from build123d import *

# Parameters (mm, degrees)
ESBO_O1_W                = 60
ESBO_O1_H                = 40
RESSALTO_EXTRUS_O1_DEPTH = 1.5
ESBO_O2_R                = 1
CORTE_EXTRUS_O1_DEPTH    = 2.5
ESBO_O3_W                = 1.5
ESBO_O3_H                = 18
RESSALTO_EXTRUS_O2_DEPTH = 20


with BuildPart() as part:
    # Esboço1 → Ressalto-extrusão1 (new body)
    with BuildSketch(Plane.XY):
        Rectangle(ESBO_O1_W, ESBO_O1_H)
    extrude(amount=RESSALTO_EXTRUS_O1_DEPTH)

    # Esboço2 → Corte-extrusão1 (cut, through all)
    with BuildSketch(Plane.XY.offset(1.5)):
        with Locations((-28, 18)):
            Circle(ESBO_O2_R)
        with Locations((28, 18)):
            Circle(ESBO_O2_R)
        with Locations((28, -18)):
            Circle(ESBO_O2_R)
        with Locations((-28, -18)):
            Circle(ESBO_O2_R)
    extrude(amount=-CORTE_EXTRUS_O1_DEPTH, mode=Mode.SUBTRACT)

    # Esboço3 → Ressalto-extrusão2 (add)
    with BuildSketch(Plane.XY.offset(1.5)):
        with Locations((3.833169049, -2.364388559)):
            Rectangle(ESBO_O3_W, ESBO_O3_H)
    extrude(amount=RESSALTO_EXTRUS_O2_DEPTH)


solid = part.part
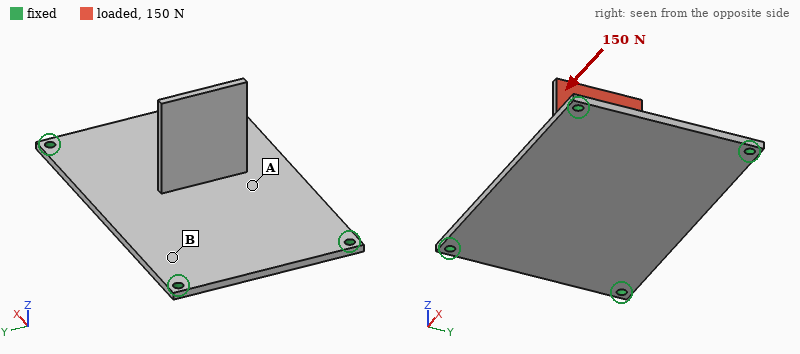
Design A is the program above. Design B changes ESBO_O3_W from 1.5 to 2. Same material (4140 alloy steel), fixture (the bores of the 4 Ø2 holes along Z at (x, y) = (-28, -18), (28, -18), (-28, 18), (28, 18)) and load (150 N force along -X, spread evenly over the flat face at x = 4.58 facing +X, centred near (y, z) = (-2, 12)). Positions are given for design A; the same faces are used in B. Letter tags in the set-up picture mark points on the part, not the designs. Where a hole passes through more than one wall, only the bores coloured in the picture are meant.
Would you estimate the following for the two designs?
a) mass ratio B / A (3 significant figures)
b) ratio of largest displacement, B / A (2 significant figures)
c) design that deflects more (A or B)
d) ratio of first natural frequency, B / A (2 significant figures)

1.04
0.61
A
0.96
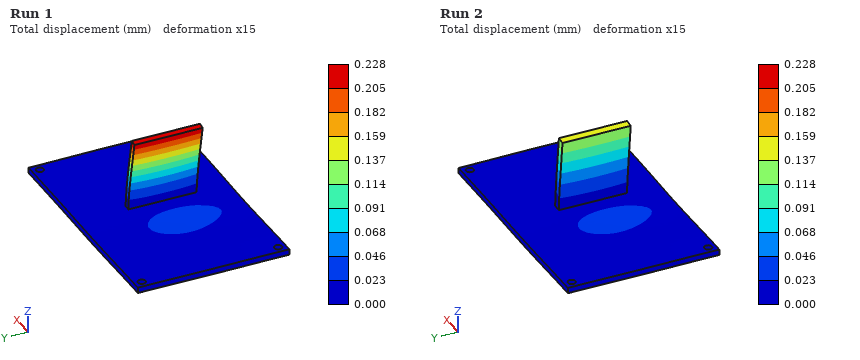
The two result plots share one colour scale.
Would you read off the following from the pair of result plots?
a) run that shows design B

Run 2
